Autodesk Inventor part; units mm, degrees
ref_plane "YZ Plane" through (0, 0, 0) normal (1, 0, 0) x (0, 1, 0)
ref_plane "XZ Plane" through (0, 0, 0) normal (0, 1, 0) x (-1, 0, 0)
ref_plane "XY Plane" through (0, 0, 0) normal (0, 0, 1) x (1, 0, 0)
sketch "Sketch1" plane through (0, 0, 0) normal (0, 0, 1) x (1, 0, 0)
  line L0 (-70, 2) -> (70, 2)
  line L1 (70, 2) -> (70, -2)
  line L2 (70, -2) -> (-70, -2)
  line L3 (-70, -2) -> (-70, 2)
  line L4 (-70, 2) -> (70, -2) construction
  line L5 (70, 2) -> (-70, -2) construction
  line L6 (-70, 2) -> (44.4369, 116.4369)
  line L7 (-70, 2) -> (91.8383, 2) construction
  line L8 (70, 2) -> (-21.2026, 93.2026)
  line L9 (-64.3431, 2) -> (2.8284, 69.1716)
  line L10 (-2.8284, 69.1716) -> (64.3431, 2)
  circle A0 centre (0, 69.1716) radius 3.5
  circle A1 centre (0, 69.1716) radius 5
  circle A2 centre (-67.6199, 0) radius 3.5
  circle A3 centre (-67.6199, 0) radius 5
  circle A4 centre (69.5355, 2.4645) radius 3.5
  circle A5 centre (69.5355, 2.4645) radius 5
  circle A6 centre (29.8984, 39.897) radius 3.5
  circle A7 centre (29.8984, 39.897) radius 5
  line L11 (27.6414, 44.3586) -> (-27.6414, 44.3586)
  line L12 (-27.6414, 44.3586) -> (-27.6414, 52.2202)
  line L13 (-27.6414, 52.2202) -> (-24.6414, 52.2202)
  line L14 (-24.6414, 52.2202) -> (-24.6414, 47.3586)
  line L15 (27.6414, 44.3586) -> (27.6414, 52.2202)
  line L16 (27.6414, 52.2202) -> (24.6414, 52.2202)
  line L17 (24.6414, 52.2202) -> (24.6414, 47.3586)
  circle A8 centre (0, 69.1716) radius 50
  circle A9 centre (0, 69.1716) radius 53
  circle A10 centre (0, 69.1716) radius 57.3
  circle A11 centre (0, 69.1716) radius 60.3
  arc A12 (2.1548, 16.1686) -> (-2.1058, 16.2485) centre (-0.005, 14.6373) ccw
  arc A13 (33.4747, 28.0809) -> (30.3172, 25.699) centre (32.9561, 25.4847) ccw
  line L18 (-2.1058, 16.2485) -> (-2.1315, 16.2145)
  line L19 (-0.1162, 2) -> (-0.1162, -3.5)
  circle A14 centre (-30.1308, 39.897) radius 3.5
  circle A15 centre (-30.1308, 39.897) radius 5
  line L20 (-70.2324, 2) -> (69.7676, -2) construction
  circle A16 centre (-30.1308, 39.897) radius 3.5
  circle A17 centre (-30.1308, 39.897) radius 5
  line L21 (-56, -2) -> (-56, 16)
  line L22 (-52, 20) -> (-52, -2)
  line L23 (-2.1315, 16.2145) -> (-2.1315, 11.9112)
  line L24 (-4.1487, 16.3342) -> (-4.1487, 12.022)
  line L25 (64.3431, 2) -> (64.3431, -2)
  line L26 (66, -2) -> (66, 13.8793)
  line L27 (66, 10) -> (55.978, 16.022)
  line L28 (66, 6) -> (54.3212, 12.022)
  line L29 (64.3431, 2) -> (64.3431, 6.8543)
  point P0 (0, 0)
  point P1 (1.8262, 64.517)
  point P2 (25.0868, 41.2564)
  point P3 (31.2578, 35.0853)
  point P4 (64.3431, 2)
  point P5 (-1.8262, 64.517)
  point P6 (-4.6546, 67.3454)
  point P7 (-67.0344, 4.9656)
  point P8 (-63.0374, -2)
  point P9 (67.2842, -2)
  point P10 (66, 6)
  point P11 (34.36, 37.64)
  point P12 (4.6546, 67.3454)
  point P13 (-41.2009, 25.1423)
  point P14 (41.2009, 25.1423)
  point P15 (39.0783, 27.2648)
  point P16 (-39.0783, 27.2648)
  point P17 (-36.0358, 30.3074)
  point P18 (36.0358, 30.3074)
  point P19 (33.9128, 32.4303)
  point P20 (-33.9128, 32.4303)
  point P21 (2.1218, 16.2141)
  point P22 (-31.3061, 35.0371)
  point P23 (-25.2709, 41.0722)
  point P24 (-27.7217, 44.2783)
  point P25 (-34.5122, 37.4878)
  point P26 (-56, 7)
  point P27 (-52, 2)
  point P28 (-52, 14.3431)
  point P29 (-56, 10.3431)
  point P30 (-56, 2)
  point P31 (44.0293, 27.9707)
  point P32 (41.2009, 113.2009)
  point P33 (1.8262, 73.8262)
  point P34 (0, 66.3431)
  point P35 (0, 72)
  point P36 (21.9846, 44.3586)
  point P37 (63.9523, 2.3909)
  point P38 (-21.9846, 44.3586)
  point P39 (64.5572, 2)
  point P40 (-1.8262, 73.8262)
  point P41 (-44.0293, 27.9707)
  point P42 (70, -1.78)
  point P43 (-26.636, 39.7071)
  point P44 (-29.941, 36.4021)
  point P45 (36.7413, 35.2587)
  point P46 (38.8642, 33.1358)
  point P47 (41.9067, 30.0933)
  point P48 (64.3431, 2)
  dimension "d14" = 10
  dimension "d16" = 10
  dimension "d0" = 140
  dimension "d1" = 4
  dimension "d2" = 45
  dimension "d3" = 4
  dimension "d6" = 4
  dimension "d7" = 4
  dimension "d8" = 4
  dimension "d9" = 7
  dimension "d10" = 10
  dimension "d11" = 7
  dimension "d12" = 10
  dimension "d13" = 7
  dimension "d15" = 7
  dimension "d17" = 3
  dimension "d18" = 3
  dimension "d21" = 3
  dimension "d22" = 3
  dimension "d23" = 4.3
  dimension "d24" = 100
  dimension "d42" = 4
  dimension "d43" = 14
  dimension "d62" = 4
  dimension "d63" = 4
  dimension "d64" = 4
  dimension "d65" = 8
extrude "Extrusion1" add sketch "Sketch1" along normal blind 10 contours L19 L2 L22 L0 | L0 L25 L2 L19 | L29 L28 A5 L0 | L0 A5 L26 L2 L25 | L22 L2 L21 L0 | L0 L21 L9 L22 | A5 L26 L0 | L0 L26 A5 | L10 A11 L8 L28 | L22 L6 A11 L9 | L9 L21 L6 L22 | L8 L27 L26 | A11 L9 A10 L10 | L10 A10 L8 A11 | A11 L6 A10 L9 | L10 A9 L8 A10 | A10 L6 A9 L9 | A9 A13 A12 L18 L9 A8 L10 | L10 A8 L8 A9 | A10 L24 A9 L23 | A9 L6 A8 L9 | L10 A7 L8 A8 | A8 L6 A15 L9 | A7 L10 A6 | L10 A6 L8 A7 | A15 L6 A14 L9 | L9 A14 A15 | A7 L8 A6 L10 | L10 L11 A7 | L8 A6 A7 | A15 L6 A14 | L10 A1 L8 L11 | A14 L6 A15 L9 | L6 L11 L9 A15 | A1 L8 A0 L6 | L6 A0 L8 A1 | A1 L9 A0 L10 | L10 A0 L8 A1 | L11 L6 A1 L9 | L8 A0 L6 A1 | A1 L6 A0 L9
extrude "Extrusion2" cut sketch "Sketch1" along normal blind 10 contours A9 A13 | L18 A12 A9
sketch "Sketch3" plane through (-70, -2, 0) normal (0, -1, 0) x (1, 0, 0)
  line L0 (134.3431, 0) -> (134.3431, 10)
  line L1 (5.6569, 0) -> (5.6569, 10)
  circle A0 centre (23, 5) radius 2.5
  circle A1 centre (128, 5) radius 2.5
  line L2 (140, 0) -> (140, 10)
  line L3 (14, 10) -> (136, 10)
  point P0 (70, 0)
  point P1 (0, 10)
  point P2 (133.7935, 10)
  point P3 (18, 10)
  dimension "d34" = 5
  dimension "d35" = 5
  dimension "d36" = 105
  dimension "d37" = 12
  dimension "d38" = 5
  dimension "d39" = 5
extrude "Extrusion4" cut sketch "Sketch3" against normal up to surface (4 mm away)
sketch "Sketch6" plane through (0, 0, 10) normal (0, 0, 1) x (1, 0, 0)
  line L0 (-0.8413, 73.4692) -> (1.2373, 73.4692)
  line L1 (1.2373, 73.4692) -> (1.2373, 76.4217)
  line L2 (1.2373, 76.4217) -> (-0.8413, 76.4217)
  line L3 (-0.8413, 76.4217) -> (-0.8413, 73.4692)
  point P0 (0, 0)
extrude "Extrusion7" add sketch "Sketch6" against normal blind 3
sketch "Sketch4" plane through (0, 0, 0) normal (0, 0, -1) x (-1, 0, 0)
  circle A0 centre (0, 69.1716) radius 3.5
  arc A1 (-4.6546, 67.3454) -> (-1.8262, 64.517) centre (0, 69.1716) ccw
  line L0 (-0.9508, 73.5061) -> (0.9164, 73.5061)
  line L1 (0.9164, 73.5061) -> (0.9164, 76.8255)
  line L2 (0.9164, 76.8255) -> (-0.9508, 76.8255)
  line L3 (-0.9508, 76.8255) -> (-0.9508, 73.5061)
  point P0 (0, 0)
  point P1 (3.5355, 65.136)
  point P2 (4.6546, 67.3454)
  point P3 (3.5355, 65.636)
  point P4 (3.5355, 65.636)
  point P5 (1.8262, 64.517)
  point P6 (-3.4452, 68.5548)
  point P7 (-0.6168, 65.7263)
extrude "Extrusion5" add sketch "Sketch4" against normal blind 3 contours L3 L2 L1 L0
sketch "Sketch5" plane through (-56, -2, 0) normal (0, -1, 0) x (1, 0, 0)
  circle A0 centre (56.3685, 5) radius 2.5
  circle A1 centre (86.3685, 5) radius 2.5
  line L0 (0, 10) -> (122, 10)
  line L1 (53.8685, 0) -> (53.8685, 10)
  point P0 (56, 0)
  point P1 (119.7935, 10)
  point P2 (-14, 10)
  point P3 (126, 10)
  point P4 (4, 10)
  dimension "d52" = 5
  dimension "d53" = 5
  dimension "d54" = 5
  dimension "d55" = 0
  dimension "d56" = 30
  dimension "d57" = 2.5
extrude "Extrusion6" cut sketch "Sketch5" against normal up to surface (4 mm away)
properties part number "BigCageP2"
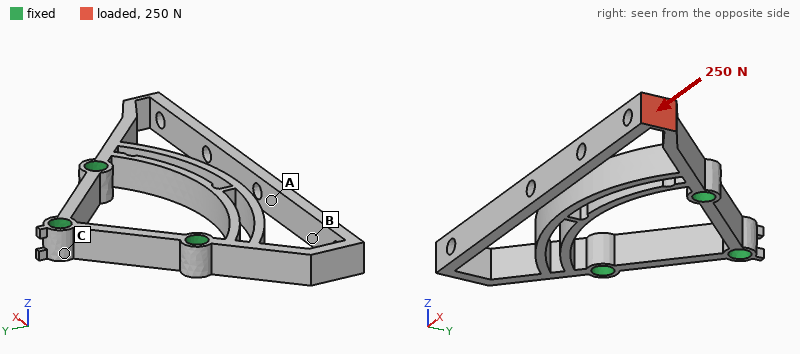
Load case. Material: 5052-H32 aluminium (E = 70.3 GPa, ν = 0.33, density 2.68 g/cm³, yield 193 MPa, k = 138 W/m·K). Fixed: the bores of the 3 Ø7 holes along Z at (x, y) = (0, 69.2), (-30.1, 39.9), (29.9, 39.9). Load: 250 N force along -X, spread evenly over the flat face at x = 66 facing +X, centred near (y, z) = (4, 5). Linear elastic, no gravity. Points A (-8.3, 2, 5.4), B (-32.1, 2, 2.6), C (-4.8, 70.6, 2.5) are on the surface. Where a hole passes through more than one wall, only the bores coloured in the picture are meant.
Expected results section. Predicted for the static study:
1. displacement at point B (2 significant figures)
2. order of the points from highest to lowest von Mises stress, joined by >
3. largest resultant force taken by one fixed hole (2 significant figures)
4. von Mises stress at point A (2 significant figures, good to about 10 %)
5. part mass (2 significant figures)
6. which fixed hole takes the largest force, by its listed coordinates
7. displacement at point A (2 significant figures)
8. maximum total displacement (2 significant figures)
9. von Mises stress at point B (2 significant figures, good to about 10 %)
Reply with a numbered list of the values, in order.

1. 0.31 mm
2. B > A > C
3. 150 N
4. 16 MPa
5. 45 g
6. (29.9, 39.9)
7. 0.36 mm
8. 0.45 mm
9. 27 MPa
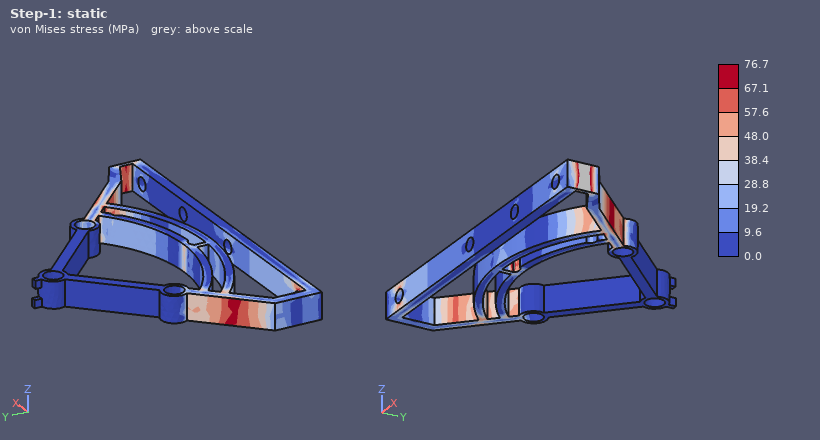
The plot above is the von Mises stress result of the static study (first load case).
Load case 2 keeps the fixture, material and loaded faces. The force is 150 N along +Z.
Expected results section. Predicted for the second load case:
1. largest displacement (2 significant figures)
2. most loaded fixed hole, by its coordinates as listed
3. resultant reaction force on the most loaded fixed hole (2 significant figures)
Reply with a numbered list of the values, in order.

1. 0.25 mm
2. (29.9, 39.9)
3. 160 N
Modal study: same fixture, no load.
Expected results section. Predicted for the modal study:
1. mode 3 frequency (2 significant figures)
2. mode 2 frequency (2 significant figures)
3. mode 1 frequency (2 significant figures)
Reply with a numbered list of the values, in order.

1. 1200 Hz
2. 1200 Hz
3. 820 Hz
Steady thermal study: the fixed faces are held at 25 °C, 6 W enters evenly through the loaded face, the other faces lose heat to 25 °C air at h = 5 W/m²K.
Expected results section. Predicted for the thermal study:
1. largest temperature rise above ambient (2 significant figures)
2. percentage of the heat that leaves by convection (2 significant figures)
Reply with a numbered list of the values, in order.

1. 40 K
2. 11 %
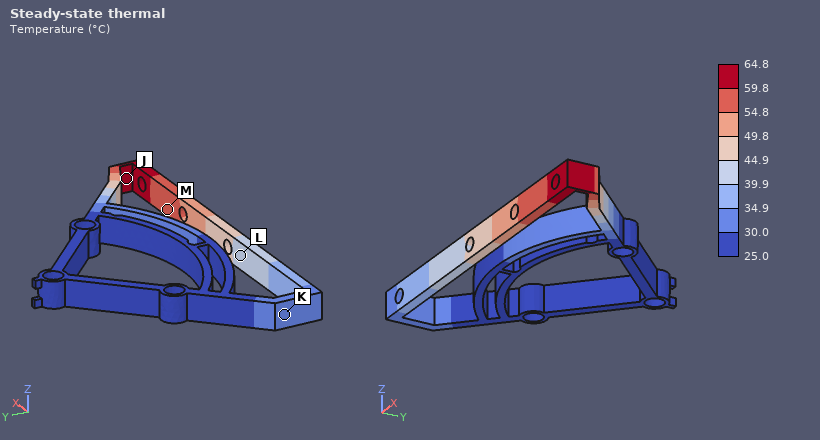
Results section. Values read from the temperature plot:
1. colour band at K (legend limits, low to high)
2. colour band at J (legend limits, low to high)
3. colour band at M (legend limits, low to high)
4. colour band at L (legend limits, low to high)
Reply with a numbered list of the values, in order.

1. 30.0 to 34.9 °C
2. 59.8 to 64.8 °C
3. 54.8 to 59.8 °C
4. 39.9 to 44.9 °C
